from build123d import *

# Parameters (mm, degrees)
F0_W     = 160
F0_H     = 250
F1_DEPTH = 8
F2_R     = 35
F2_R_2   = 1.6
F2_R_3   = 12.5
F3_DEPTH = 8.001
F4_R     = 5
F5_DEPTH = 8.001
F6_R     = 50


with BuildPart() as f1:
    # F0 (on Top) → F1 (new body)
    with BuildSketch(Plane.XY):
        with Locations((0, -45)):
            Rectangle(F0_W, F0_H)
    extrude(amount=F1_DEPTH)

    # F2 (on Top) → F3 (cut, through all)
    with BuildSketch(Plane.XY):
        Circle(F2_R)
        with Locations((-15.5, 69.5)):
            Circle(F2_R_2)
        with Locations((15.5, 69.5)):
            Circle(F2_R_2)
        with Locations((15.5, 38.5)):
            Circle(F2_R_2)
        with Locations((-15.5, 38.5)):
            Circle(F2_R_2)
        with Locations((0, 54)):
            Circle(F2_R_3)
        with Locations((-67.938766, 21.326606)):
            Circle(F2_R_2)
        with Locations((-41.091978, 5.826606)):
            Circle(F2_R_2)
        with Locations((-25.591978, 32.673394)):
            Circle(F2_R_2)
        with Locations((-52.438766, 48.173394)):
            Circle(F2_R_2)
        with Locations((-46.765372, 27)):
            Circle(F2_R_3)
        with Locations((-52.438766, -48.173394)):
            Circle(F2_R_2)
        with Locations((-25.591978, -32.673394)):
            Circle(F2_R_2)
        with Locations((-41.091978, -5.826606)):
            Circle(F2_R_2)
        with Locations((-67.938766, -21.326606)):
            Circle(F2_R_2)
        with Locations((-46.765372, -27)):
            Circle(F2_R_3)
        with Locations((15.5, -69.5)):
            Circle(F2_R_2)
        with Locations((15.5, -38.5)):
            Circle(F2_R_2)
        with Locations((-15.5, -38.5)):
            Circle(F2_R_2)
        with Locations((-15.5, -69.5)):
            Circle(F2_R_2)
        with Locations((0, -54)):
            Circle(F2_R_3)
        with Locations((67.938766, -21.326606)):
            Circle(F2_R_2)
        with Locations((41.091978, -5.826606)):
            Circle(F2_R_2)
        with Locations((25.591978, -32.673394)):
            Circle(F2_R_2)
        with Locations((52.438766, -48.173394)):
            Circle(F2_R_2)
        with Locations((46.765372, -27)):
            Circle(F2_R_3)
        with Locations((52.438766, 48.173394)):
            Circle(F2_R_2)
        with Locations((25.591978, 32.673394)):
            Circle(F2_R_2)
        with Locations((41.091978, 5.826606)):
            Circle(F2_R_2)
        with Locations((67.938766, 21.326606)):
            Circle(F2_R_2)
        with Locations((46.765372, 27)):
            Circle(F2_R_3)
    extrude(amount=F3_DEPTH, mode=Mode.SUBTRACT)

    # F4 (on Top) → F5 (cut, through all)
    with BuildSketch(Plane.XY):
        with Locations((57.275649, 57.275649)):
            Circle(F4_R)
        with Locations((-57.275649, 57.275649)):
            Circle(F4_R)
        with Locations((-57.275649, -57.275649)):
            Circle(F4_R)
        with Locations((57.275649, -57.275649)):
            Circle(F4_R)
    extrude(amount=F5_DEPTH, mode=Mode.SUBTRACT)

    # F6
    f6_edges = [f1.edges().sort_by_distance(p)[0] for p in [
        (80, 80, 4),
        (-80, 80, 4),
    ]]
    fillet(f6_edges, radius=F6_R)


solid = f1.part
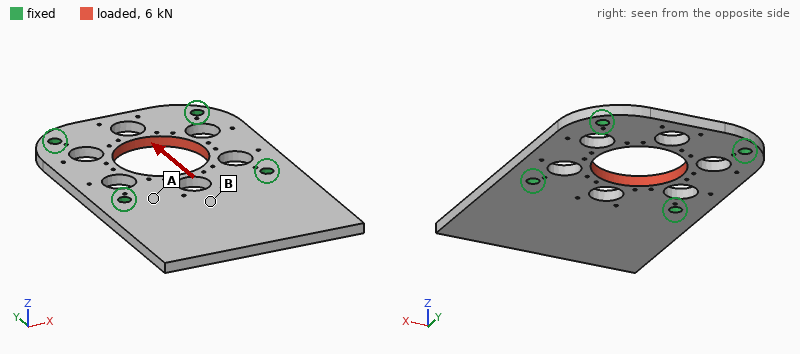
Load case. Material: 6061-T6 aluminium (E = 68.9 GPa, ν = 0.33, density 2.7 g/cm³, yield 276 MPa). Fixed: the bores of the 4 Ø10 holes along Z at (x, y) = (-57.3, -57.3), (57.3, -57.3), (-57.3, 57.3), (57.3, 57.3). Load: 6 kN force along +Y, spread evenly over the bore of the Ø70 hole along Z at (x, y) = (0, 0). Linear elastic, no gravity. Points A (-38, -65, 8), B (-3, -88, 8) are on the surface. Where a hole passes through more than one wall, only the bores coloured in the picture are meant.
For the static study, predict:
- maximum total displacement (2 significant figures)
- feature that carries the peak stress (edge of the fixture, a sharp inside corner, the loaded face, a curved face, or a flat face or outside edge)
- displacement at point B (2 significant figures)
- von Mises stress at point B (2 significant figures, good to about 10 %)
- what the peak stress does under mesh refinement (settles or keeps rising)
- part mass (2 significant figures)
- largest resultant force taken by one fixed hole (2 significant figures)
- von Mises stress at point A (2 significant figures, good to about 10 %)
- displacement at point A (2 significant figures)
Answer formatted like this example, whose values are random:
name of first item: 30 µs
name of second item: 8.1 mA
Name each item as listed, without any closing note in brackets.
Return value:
maximum total displacement: 12 µm
feature that carries the peak stress: edge of the fixture
displacement at point B: 2.8 µm
von Mises stress at point B: 1.3 MPa
what the peak stress does under mesh refinement: keeps rising
part mass: 680 g
largest resultant force taken by one fixed hole: 1.6 kN
von Mises stress at point A: 3.9 MPa
displacement at point A: 2.3 µm
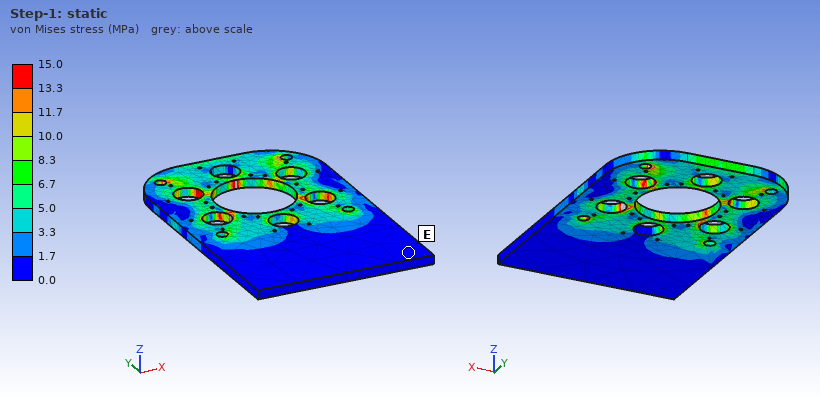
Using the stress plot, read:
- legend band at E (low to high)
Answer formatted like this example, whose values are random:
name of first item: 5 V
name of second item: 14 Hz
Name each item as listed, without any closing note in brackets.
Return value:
legend band at E: 0.0 to 1.7 MPa
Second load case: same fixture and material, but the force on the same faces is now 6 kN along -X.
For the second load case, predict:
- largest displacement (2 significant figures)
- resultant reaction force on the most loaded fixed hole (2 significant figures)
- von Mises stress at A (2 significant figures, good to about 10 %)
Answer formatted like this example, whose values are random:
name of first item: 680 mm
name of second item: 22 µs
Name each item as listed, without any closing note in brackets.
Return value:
largest displacement: 13 µm
resultant reaction force on the most loaded fixed hole: 1.6 kN
von Mises stress at A: 1.5 MPa
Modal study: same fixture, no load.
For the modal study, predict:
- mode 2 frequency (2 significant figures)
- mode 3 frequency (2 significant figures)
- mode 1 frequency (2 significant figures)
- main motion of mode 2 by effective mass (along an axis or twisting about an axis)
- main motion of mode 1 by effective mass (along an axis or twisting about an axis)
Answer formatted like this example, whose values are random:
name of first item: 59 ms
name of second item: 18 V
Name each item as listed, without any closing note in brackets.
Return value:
mode 2 frequency: 990 Hz
mode 3 frequency: 2200 Hz
mode 1 frequency: 470 Hz
main motion of mode 2 by effective mass: twisting about Y
main motion of mode 1 by effective mass: along Z
